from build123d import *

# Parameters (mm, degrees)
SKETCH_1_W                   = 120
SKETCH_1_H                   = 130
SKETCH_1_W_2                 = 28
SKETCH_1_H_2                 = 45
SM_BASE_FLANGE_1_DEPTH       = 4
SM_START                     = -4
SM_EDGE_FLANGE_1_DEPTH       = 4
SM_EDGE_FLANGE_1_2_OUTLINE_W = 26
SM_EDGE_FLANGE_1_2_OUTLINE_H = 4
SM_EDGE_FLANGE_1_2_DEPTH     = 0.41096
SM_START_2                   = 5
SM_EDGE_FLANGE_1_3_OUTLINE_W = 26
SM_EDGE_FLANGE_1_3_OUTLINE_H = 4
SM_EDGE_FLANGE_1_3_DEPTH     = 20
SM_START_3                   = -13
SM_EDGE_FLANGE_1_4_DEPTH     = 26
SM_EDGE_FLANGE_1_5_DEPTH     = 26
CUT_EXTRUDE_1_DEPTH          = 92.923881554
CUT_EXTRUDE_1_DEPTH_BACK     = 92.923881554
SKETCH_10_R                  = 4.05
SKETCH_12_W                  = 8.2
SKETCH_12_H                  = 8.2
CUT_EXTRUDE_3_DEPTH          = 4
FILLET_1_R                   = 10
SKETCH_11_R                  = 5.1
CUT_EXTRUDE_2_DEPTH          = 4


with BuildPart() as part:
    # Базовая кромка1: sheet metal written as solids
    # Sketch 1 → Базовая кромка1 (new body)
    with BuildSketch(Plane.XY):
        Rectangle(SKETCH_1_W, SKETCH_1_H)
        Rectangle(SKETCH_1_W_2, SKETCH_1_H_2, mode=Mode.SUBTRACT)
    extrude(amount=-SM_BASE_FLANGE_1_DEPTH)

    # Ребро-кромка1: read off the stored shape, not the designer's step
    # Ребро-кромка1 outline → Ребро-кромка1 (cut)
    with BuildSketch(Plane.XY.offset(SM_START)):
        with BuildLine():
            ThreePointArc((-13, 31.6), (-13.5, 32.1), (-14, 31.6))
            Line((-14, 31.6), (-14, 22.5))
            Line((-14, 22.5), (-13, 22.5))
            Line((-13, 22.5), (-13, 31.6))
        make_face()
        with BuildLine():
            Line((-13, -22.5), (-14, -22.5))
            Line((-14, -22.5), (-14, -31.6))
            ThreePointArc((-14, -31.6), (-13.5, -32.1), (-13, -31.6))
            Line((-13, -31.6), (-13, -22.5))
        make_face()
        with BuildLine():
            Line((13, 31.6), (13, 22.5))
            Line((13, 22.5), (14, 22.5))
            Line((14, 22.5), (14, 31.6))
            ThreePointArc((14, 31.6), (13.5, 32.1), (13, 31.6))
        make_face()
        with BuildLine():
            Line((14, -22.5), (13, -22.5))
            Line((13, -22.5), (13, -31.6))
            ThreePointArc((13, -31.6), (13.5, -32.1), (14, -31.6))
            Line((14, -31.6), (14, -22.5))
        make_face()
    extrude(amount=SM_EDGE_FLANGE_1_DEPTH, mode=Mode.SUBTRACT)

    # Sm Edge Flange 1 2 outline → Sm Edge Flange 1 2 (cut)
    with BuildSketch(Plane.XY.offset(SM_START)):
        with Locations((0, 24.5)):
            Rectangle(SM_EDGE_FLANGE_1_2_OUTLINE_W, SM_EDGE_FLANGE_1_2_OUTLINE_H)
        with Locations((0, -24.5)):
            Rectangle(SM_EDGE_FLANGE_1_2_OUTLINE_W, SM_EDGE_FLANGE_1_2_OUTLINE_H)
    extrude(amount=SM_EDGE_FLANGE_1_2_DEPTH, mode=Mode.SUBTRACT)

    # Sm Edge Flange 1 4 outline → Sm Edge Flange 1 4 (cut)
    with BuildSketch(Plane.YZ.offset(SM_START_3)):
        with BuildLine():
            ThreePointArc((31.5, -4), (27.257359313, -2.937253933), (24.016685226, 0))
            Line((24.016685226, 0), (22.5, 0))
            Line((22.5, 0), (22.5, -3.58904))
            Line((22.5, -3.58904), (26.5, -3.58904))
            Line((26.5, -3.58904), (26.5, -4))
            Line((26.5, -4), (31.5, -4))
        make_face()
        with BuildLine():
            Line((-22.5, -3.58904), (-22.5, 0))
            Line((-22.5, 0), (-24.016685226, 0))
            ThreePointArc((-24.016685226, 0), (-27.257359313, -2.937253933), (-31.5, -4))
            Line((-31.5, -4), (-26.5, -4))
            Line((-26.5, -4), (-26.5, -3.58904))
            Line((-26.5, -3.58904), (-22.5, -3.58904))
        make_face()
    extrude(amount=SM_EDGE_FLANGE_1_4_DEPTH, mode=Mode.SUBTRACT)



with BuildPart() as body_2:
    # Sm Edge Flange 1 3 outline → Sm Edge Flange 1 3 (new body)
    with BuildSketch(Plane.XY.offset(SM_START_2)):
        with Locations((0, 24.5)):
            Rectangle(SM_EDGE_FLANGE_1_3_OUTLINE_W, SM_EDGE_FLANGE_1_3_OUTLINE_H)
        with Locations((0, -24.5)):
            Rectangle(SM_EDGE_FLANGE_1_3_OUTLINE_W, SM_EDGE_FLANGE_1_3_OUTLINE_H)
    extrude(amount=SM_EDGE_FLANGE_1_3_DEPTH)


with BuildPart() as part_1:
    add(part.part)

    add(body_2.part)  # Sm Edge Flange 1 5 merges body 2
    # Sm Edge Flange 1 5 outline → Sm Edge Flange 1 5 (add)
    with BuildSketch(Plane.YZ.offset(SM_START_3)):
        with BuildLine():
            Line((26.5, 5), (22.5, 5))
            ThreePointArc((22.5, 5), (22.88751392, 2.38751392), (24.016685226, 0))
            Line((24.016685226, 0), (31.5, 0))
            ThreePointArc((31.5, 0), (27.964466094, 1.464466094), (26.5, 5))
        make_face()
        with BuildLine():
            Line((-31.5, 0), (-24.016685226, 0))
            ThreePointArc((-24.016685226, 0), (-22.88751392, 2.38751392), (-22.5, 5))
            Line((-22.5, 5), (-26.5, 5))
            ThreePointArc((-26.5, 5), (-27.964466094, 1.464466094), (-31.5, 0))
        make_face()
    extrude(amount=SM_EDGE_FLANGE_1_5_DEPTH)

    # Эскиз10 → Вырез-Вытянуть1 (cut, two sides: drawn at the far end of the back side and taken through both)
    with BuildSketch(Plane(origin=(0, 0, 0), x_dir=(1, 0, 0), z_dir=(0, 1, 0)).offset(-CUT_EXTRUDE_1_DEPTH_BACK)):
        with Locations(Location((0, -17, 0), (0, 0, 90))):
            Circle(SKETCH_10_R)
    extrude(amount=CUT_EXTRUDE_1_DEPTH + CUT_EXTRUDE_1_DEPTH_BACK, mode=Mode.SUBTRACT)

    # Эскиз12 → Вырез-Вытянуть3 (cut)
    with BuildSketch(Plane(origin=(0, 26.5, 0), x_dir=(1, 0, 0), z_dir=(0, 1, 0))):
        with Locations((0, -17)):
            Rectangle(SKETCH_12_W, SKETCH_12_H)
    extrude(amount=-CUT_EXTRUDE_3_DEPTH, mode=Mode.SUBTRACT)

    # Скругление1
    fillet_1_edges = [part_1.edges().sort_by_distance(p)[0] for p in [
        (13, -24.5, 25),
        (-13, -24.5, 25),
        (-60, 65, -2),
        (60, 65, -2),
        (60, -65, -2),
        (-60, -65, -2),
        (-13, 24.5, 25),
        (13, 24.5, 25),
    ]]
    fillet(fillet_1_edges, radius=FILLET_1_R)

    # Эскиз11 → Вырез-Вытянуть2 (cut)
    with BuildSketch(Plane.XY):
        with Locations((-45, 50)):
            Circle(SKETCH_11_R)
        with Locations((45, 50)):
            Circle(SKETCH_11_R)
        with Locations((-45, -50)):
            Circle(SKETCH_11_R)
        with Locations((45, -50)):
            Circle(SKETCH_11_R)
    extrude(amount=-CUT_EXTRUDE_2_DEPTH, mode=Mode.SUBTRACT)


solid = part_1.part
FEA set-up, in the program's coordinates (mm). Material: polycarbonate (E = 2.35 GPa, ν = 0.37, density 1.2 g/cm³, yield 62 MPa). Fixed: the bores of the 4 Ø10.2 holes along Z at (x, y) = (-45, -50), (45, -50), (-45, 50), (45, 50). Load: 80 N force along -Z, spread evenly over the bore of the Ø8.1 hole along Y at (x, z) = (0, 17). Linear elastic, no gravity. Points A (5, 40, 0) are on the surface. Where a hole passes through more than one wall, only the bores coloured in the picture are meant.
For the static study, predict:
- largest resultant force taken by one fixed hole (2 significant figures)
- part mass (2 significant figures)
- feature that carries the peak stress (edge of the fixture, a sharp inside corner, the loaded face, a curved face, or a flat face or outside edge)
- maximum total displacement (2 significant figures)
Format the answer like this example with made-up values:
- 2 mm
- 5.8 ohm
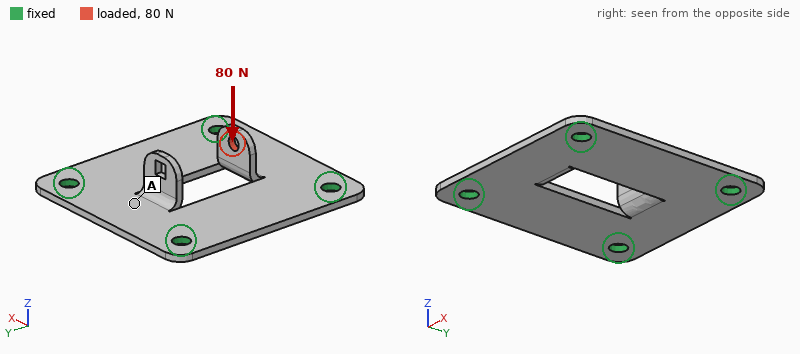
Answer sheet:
- 34 N
- 71 g
- a curved face
- 1.8 mm
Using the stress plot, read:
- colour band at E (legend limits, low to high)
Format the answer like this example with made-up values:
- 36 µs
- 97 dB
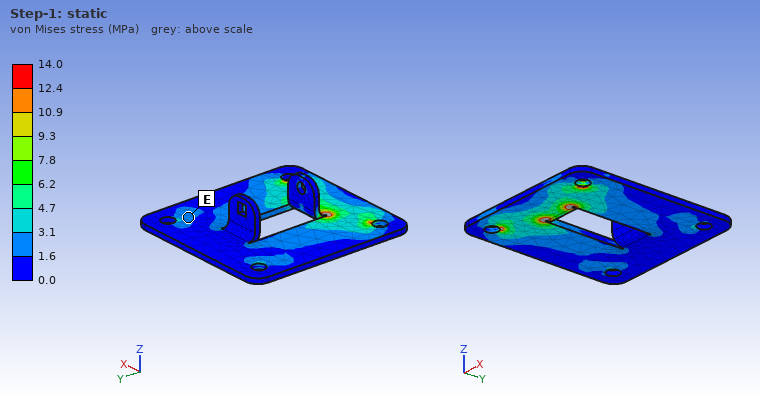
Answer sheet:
- 1.6 to 3.1 MPa
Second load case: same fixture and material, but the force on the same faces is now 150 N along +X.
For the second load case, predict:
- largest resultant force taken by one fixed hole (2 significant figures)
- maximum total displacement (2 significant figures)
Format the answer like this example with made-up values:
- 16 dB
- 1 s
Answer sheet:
- 98 N
- 1.7 mm
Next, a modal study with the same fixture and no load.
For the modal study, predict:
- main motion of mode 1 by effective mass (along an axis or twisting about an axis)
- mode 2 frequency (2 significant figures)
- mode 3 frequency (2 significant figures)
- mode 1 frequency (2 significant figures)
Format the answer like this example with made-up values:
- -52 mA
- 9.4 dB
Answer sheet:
- along Z
- 620 Hz
- 650 Hz
- 430 Hz
